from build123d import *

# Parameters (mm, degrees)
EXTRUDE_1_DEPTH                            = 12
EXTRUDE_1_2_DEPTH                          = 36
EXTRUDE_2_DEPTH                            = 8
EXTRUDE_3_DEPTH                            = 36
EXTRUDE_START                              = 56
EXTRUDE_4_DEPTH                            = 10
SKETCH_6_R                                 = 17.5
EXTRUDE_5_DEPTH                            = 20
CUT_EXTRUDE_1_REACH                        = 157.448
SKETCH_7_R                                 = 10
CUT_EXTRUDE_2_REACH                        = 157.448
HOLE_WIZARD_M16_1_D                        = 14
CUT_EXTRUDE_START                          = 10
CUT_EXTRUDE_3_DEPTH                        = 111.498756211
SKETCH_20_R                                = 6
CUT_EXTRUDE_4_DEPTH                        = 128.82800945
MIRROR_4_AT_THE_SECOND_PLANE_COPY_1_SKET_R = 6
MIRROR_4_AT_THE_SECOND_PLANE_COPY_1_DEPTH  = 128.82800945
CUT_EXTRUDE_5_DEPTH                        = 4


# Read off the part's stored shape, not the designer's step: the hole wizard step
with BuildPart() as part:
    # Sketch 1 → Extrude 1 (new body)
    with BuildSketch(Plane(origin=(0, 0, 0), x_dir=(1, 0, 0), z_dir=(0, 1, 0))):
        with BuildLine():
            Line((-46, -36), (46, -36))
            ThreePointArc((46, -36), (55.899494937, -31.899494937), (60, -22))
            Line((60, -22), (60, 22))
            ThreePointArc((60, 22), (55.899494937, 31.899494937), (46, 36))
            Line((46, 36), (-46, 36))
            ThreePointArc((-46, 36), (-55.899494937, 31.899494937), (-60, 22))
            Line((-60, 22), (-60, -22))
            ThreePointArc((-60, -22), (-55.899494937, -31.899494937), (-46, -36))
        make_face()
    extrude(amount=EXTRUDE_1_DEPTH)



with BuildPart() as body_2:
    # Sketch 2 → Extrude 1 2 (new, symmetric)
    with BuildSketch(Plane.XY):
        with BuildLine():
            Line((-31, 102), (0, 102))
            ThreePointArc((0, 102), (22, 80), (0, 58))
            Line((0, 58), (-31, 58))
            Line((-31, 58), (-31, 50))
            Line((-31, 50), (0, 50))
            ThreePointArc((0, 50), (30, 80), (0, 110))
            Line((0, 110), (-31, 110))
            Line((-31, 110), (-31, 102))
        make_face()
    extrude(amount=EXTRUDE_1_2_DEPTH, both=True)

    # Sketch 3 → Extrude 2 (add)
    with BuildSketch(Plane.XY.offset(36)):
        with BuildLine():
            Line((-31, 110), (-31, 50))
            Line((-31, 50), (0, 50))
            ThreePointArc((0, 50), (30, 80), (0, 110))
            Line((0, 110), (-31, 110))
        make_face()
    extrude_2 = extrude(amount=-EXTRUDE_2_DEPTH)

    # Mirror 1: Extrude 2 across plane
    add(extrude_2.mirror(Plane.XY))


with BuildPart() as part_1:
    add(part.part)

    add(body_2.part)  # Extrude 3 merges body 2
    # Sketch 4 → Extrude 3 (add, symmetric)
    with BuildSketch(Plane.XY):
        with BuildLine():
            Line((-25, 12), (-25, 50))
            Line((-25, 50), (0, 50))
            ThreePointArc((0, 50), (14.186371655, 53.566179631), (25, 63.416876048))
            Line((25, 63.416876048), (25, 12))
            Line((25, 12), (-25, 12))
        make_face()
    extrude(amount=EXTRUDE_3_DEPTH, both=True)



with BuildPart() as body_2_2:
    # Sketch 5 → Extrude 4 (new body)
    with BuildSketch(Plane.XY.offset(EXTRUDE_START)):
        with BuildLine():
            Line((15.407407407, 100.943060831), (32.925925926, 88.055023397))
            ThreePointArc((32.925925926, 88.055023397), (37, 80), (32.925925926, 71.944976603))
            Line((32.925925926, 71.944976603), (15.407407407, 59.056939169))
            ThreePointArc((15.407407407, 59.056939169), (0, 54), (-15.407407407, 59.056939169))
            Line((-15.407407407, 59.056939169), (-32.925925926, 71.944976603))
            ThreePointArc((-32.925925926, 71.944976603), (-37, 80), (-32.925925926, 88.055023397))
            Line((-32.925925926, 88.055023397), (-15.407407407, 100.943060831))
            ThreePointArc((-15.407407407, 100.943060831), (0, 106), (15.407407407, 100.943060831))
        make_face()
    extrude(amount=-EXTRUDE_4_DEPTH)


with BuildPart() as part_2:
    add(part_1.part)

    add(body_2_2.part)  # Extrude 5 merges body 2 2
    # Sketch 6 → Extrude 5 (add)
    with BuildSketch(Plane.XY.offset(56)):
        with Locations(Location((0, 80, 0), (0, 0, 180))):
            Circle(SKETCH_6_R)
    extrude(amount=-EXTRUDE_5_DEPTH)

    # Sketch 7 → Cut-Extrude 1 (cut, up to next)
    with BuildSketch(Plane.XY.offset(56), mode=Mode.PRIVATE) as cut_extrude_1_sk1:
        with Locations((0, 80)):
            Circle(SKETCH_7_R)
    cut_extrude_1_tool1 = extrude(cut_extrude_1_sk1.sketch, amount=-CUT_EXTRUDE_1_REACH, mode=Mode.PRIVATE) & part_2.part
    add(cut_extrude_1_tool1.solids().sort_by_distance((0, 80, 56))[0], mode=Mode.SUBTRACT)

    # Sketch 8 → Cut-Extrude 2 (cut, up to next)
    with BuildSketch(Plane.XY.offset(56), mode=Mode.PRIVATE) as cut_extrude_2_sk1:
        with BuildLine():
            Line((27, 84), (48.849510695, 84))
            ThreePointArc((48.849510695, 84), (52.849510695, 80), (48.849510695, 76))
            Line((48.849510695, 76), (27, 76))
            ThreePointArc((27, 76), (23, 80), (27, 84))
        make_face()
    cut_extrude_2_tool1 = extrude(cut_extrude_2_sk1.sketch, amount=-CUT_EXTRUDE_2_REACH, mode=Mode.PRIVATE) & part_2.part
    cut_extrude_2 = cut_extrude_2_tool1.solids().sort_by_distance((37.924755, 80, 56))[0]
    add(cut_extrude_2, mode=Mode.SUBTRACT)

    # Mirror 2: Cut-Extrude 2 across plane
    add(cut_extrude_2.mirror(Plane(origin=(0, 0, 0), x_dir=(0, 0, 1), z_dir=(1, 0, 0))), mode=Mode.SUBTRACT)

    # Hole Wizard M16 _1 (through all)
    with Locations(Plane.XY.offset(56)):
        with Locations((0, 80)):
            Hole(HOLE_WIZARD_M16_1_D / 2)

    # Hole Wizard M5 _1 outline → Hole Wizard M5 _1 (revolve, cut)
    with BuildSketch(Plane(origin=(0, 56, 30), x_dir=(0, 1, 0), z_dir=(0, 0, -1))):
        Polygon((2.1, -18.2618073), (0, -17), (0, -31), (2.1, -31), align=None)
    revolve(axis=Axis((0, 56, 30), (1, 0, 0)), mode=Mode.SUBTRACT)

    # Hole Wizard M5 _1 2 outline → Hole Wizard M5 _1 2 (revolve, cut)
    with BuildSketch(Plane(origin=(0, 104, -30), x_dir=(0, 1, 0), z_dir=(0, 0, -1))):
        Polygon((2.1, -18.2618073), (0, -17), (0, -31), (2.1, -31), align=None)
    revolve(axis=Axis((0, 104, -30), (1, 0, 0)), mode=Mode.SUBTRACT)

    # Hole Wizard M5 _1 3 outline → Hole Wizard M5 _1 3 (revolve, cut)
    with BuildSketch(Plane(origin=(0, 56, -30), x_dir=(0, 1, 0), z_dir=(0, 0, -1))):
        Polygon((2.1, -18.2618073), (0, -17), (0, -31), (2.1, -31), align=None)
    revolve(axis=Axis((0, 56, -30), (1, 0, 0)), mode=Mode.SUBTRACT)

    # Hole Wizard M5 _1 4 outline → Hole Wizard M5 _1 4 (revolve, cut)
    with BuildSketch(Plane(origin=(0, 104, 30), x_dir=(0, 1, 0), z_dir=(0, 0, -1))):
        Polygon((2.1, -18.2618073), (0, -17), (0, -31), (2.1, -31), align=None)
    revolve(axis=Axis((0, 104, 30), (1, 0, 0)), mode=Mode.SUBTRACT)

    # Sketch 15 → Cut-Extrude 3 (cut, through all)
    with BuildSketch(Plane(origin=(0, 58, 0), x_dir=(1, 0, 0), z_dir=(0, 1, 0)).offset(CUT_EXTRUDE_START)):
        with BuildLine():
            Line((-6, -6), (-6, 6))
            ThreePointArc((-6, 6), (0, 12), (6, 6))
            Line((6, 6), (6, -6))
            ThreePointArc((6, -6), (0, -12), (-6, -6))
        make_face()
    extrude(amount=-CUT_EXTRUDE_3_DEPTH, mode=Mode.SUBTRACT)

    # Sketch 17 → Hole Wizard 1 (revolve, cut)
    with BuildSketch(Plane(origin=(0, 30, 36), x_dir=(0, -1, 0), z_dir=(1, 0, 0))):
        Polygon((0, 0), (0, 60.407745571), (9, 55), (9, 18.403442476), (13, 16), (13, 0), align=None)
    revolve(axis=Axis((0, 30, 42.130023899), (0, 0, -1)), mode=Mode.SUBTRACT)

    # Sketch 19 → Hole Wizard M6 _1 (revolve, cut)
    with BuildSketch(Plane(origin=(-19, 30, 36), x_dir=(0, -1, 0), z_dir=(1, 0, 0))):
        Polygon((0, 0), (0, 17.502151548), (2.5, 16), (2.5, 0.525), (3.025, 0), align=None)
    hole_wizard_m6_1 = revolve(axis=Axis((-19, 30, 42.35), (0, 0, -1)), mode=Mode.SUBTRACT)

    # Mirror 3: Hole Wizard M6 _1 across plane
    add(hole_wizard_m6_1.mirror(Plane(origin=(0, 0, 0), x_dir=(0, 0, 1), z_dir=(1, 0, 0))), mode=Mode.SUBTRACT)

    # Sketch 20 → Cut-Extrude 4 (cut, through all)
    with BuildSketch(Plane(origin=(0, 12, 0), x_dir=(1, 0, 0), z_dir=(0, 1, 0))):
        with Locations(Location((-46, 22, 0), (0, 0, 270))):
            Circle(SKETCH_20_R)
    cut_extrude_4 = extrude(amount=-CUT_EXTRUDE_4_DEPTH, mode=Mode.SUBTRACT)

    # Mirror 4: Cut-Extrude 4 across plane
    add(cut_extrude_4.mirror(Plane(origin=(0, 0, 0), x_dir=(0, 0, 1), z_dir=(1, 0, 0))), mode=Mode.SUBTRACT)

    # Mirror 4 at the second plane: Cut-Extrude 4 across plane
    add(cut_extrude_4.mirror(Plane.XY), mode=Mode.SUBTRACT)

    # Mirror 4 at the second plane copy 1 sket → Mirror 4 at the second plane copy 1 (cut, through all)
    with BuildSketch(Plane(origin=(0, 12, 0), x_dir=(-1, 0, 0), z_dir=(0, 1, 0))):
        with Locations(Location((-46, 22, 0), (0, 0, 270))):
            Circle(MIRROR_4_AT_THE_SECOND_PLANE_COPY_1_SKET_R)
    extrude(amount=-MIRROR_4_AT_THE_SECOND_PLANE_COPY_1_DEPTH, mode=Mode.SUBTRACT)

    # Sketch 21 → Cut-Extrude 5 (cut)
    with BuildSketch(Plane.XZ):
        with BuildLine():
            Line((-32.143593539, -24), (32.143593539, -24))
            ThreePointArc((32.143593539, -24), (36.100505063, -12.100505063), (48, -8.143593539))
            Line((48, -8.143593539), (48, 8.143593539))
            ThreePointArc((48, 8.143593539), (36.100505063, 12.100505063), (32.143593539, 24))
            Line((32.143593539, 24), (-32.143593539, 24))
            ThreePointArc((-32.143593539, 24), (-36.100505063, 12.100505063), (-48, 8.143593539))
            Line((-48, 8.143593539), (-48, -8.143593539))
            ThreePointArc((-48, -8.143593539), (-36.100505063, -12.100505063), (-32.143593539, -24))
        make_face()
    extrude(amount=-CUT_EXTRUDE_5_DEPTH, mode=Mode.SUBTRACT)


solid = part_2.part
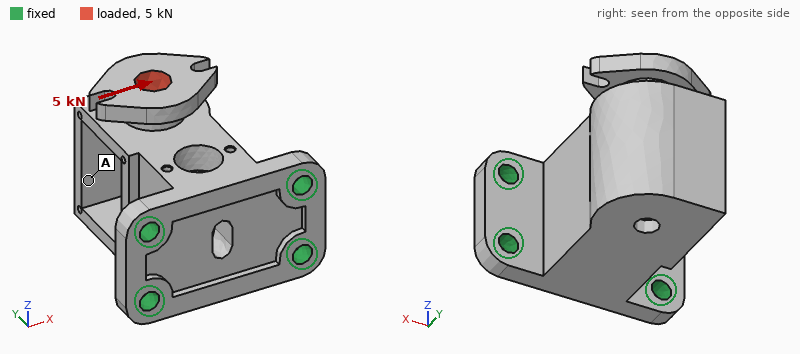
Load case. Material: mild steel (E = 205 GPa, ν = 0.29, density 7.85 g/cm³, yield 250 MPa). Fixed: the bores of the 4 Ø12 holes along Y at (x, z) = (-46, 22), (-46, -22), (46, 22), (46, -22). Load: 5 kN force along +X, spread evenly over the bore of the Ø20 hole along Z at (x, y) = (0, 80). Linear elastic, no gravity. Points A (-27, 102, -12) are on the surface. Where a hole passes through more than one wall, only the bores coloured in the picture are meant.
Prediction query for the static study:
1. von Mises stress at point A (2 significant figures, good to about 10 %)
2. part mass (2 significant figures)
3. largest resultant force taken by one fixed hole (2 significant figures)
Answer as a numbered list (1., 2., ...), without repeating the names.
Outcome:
1. 5.3 MPa
2. 2.6 kg
3. 3.5 kN
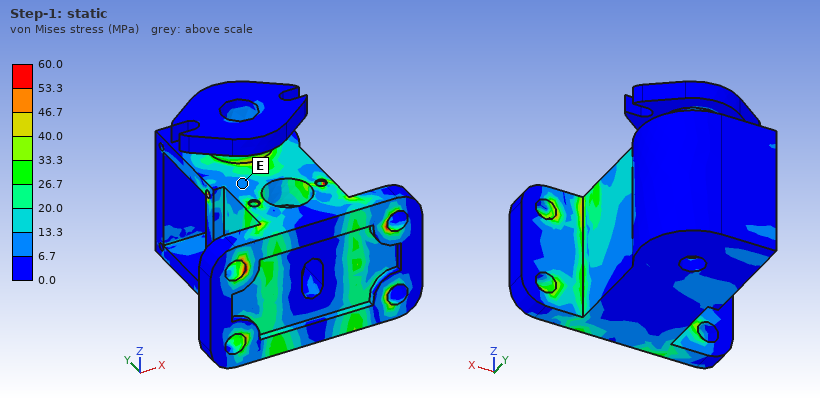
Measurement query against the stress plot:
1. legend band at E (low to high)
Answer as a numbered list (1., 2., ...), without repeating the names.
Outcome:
1. 6.7 to 13.3 MPa
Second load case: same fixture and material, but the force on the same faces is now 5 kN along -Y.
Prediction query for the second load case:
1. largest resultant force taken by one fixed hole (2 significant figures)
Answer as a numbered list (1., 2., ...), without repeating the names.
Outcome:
1. 3.6 kN
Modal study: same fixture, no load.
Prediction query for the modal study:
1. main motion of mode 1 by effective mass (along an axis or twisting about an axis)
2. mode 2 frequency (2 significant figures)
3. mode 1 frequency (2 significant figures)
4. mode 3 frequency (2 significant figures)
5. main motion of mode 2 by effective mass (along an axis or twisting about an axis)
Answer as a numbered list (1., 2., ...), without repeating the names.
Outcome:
1. along Z
2. 2000 Hz
3. 1500 Hz
4. 3700 Hz
5. along X
